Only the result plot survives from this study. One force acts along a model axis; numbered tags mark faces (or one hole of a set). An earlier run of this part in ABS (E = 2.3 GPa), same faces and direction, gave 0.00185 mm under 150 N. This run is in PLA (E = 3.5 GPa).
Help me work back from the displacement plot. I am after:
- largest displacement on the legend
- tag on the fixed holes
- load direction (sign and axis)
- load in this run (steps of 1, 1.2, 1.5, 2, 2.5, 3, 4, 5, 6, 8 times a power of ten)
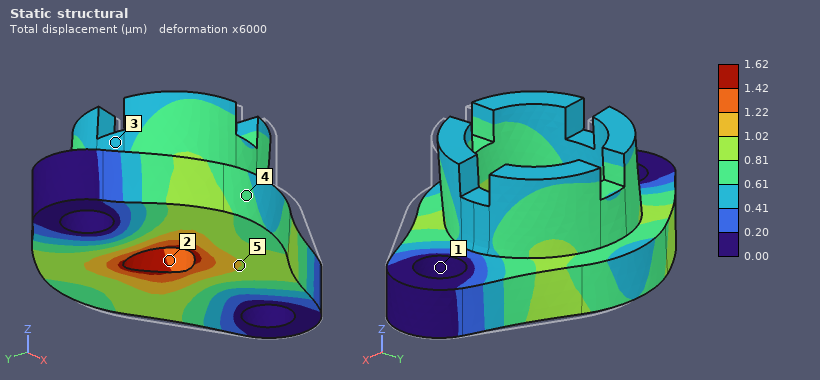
1.62 µm
1
-X
200 N
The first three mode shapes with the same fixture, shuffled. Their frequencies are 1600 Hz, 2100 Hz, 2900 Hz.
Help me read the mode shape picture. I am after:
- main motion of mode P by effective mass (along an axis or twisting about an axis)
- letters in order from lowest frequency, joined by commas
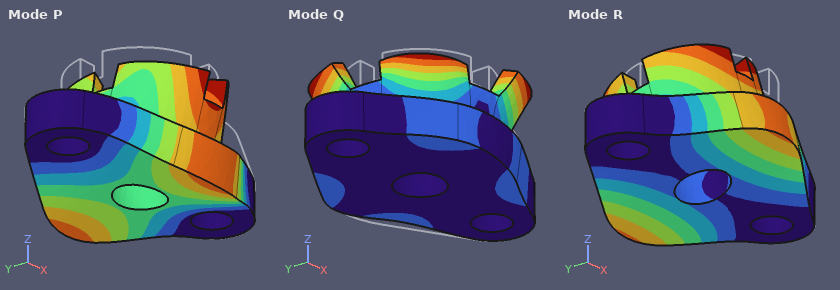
along Z
R, P, Q
